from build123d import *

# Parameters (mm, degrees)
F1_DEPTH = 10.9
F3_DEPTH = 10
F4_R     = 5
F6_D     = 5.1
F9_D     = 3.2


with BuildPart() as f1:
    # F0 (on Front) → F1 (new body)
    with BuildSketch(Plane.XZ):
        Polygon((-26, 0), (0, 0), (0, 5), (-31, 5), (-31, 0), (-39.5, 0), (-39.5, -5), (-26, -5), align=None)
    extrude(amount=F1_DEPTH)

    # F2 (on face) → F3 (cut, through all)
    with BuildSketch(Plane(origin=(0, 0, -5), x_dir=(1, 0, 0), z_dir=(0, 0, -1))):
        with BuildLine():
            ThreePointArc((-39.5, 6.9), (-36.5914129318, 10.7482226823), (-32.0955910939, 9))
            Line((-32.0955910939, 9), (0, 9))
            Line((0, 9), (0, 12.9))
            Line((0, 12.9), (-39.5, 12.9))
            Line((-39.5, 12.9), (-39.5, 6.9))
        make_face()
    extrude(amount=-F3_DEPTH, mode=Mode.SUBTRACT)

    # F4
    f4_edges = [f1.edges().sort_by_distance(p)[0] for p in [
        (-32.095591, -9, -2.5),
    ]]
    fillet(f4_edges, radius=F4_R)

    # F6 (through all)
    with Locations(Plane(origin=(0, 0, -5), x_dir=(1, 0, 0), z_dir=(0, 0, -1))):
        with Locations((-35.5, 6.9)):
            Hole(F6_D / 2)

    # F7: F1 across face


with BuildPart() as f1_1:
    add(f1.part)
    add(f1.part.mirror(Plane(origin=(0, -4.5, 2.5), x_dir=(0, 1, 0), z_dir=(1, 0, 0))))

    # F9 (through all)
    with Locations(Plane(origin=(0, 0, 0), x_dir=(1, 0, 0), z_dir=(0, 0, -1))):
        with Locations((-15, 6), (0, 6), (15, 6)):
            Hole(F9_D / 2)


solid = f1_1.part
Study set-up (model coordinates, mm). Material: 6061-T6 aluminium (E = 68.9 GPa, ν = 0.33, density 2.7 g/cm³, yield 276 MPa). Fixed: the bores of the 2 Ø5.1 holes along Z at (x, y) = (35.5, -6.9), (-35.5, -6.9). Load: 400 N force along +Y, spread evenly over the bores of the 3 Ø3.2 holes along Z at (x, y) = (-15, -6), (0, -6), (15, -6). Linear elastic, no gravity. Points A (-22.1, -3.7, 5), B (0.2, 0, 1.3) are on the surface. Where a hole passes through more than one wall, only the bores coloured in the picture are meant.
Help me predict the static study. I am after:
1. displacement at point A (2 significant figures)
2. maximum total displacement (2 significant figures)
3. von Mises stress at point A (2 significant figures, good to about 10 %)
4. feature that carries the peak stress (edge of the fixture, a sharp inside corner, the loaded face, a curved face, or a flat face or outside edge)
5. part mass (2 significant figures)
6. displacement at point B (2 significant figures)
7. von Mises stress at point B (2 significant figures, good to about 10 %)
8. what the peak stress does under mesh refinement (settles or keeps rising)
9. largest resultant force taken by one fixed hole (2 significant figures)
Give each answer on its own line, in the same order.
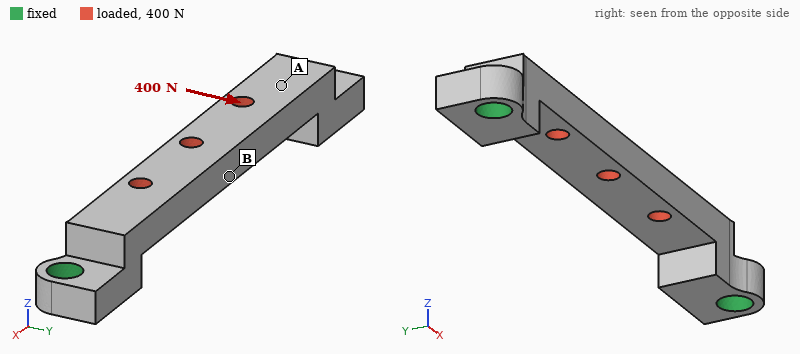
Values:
16 µm
39 µm
9.5 MPa
a sharp inside corner
10 g
38 µm
34 MPa
keeps rising
210 N
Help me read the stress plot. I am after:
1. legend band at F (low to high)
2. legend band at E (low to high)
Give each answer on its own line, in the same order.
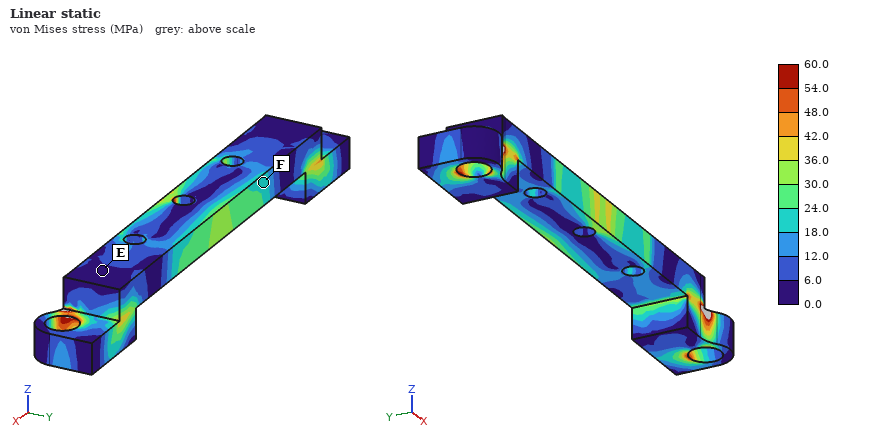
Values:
18.0 to 24.0 MPa
0.0 to 6.0 MPa
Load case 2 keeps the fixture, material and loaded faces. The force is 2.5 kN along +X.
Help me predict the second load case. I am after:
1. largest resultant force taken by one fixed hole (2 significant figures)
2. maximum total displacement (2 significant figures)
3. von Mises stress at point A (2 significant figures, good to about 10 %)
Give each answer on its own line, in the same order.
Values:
1.3 kN
38 µm
21 MPa
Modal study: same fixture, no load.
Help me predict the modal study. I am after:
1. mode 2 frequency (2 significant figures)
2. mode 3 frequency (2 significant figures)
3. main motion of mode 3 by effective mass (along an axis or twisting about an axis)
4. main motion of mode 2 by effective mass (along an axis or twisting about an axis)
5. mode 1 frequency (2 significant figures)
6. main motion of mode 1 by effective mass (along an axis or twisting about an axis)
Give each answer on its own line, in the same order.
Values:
7900 Hz
12 kHz
along X
along Y
6300 Hz
along Z
